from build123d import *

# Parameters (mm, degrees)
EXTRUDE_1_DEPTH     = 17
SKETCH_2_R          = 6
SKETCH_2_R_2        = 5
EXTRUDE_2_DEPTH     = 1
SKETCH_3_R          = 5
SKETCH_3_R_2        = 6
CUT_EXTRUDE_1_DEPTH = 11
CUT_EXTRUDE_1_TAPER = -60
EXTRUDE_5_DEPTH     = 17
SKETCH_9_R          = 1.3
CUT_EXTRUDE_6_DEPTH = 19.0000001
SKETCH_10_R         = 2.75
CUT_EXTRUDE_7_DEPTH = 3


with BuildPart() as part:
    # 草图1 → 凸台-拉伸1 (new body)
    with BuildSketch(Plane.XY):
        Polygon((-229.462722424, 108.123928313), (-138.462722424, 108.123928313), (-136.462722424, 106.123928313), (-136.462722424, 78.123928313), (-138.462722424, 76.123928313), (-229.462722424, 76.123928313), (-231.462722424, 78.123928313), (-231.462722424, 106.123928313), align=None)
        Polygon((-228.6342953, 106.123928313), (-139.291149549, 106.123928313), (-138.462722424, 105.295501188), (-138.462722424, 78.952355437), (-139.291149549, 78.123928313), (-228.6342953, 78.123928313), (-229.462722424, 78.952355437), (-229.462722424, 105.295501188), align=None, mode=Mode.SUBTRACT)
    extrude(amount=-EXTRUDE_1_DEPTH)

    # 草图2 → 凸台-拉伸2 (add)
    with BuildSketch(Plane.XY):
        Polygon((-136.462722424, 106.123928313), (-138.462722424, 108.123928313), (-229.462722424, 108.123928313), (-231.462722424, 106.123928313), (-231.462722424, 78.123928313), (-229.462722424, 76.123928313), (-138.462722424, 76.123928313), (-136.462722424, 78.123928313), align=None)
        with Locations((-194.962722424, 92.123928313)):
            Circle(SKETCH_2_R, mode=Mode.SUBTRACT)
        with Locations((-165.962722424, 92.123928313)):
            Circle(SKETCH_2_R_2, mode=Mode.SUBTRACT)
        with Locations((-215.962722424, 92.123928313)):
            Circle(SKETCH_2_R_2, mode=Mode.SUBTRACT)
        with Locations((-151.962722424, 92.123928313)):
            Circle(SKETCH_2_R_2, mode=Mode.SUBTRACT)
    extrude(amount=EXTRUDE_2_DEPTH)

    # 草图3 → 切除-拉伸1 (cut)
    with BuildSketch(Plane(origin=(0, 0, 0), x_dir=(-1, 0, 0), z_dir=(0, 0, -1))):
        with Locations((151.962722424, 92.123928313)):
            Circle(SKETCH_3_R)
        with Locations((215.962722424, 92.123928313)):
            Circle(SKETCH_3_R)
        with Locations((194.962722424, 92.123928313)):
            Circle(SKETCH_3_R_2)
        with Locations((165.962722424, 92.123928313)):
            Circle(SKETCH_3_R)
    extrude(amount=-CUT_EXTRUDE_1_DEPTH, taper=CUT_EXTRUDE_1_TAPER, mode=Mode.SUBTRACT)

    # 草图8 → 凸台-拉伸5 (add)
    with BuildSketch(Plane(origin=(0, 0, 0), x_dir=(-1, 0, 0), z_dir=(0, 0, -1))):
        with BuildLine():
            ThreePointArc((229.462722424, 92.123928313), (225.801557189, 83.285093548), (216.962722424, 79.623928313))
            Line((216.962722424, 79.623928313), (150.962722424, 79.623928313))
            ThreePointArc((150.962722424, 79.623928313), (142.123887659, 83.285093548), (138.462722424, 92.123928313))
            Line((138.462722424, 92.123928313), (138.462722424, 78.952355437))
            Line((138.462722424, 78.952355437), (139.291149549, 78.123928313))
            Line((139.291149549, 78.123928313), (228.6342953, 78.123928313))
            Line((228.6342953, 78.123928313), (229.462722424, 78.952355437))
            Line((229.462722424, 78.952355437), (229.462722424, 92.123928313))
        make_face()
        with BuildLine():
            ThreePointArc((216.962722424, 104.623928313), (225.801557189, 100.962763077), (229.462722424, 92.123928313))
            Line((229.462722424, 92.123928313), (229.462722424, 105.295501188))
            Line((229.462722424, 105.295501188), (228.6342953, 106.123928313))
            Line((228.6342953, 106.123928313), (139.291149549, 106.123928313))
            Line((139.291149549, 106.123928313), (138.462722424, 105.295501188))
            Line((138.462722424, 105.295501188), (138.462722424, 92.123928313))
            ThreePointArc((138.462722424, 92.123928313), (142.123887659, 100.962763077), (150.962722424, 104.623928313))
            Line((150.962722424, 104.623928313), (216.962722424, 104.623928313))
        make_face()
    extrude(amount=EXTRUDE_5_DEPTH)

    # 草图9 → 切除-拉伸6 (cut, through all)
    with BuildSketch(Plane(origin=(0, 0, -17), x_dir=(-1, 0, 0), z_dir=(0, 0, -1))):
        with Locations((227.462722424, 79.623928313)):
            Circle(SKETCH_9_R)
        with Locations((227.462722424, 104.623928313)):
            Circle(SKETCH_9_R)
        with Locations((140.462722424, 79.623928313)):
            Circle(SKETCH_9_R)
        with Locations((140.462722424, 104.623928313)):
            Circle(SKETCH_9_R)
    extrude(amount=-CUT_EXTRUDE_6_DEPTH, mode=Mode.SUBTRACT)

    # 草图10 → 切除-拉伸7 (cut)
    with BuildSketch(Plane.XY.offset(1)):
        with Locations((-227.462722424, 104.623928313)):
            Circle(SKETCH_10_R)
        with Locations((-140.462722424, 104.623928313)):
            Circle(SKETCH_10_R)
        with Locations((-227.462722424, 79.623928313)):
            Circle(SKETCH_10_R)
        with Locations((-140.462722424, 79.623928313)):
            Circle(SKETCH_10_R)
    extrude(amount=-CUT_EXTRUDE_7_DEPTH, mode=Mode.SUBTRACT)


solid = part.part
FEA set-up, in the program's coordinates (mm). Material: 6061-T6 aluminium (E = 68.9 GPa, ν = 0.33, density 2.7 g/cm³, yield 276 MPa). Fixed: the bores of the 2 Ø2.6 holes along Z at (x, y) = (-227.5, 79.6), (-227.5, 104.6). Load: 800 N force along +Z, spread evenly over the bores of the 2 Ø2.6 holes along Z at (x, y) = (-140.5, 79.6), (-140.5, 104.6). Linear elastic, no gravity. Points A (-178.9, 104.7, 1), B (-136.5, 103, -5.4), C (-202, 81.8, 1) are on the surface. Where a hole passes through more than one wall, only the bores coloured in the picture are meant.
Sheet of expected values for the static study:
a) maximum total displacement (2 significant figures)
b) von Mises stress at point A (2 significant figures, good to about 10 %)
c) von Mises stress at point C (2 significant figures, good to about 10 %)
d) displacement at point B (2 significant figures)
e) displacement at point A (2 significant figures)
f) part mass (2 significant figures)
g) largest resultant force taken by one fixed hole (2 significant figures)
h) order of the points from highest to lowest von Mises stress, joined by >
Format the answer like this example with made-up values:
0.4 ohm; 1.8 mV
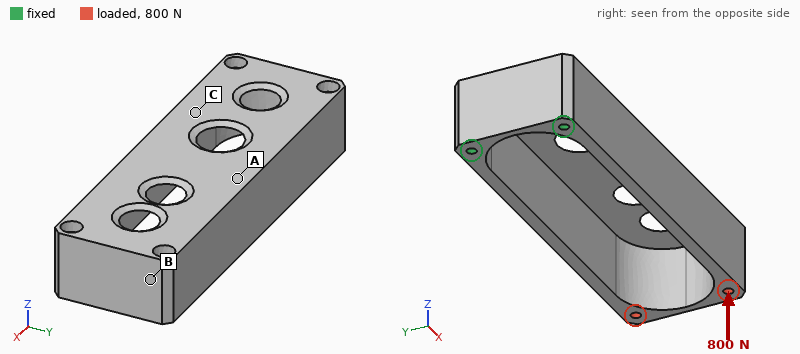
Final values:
0.70 mm; 55 MPa; 94 MPa; 0.69 mm; 0.27 mm; 46 g; 430 N; C > A > B
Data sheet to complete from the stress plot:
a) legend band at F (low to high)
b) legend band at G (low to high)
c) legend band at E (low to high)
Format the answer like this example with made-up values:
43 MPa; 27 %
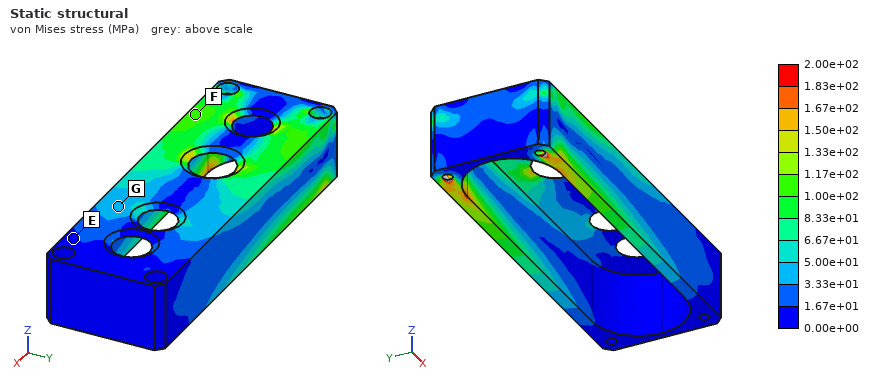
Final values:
1.00e+02 to 1.17e+02 MPa; 3.33e+01 to 5.00e+01 MPa; 0.00e+00 to 1.67e+01 MPa
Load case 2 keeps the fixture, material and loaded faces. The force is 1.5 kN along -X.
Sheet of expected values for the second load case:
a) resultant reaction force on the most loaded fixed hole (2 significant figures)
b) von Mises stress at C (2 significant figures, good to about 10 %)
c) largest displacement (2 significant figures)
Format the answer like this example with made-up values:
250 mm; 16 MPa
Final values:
750 N; 4.3 MPa; 56 µm
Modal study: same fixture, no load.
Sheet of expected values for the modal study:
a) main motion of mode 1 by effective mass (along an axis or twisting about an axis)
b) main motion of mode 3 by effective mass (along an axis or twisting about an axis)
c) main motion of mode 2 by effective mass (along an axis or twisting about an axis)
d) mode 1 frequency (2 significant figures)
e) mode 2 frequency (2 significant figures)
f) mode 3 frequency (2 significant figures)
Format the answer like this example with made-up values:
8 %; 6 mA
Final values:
along Y; along Y; along Z; 1300 Hz; 1400 Hz; 3600 Hz
